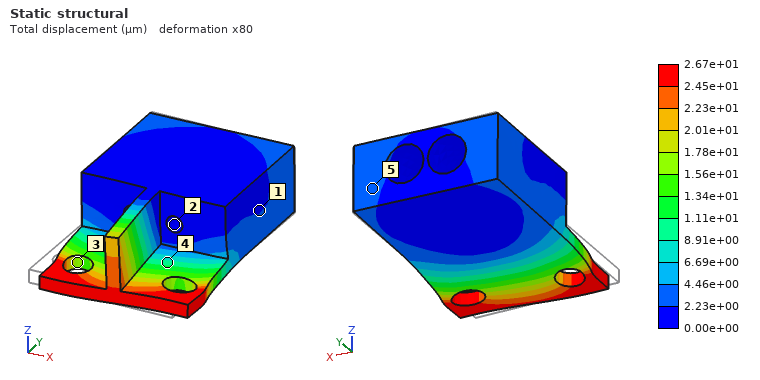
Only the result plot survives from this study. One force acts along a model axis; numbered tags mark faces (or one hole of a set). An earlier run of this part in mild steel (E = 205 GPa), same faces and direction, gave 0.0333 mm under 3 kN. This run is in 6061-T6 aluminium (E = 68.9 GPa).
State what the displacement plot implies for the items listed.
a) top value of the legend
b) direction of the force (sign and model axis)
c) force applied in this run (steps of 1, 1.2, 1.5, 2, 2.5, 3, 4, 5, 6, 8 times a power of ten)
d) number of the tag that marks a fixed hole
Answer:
2.67e+01 µm
+X
800 N
2
